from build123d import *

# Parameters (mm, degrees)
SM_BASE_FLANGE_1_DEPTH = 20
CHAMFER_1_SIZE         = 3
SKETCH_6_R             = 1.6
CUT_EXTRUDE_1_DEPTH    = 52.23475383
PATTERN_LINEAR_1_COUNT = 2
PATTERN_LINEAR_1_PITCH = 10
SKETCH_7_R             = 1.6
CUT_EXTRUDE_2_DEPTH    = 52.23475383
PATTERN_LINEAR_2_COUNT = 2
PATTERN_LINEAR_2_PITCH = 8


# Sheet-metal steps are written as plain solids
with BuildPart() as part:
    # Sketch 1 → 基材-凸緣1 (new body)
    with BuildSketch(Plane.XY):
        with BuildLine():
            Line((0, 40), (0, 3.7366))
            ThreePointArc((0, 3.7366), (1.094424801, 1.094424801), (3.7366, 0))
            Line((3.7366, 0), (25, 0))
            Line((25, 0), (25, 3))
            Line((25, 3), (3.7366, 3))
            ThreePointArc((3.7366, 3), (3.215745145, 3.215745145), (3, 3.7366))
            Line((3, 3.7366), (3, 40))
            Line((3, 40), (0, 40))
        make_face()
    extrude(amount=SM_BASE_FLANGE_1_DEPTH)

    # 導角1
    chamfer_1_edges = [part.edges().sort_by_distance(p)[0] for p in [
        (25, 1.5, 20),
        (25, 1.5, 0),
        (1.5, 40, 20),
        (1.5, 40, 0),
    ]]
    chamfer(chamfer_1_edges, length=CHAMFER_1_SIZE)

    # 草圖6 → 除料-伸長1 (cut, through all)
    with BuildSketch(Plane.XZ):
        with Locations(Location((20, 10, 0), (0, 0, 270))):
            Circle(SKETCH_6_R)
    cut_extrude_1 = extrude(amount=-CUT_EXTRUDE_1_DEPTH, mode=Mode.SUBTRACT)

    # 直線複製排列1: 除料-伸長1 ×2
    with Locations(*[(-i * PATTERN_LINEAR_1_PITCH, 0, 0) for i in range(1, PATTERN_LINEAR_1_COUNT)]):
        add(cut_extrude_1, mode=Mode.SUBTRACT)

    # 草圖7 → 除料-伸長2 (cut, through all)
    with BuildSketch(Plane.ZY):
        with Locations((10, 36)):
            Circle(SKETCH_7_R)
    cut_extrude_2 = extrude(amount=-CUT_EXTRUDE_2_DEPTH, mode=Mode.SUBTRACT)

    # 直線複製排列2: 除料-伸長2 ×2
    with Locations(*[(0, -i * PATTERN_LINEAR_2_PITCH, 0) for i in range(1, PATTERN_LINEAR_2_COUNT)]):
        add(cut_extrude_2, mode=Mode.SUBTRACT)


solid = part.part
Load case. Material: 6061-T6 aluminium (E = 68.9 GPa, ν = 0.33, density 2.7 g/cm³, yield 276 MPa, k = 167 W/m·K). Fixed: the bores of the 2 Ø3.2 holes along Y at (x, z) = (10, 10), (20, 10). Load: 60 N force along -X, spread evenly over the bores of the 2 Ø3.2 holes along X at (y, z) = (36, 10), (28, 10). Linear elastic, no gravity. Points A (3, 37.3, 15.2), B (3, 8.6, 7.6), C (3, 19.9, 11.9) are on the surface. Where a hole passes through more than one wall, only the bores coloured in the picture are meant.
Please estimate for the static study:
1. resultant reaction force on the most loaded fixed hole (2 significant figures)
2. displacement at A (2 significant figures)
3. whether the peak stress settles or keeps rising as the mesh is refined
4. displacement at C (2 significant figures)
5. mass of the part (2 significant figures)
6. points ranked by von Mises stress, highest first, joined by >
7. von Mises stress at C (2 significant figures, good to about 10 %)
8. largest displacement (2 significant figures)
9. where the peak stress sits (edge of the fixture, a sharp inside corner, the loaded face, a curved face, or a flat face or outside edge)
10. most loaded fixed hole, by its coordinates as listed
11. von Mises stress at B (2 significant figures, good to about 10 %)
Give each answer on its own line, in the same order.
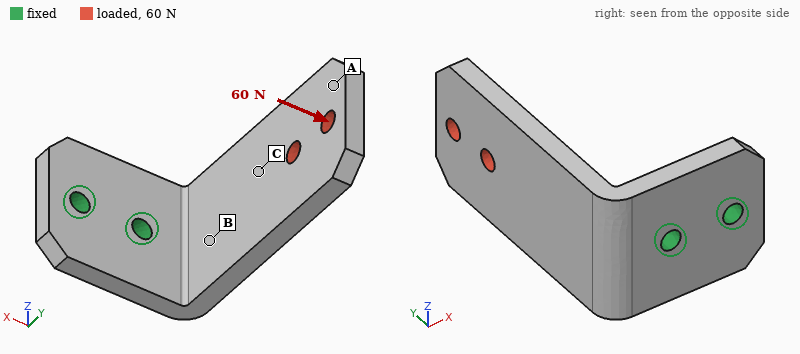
90 N
0.38 mm
keeps rising
0.16 mm
9.5 g
B > C > A
24 MPa
0.42 mm
edge of the fixture
(10, 10)
43 MPa
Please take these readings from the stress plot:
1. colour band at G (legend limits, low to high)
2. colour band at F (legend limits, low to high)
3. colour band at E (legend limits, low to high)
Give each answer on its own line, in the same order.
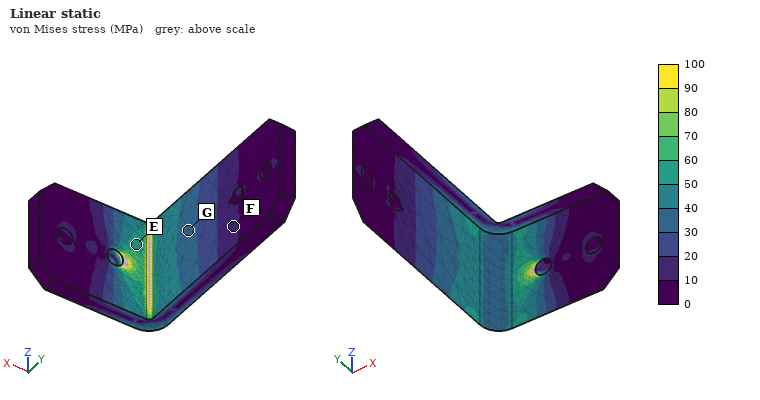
30 to 40 MPa
10 to 20 MPa
50 to 60 MPa
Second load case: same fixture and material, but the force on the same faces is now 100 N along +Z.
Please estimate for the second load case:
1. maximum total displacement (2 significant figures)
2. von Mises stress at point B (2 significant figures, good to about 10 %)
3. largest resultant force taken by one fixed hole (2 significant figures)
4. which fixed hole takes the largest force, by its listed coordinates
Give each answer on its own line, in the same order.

0.20 mm
17 MPa
160 N
(10, 10)
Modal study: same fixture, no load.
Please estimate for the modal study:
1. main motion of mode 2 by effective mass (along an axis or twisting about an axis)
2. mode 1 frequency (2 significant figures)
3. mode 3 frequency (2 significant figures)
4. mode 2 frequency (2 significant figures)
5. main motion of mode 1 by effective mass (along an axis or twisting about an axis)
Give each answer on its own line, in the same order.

along Z
1300 Hz
6300 Hz
2200 Hz
along X
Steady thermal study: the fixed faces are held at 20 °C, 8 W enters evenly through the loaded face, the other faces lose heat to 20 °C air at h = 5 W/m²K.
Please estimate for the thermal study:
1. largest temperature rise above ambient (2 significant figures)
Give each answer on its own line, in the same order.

33 K
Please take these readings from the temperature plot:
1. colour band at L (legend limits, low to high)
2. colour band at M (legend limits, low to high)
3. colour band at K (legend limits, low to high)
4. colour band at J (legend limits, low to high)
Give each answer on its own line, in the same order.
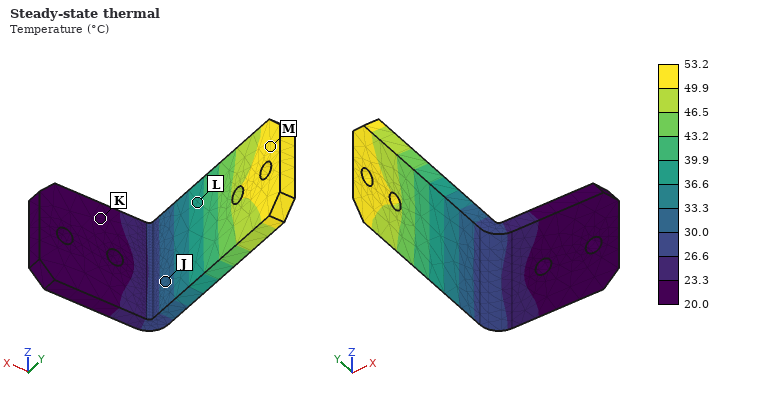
36.6 to 39.9 °C
49.9 to 53.2 °C
20.0 to 23.3 °C
30.0 to 33.3 °C
